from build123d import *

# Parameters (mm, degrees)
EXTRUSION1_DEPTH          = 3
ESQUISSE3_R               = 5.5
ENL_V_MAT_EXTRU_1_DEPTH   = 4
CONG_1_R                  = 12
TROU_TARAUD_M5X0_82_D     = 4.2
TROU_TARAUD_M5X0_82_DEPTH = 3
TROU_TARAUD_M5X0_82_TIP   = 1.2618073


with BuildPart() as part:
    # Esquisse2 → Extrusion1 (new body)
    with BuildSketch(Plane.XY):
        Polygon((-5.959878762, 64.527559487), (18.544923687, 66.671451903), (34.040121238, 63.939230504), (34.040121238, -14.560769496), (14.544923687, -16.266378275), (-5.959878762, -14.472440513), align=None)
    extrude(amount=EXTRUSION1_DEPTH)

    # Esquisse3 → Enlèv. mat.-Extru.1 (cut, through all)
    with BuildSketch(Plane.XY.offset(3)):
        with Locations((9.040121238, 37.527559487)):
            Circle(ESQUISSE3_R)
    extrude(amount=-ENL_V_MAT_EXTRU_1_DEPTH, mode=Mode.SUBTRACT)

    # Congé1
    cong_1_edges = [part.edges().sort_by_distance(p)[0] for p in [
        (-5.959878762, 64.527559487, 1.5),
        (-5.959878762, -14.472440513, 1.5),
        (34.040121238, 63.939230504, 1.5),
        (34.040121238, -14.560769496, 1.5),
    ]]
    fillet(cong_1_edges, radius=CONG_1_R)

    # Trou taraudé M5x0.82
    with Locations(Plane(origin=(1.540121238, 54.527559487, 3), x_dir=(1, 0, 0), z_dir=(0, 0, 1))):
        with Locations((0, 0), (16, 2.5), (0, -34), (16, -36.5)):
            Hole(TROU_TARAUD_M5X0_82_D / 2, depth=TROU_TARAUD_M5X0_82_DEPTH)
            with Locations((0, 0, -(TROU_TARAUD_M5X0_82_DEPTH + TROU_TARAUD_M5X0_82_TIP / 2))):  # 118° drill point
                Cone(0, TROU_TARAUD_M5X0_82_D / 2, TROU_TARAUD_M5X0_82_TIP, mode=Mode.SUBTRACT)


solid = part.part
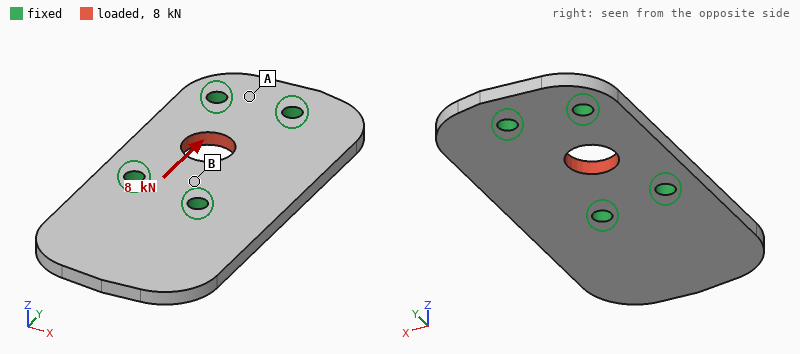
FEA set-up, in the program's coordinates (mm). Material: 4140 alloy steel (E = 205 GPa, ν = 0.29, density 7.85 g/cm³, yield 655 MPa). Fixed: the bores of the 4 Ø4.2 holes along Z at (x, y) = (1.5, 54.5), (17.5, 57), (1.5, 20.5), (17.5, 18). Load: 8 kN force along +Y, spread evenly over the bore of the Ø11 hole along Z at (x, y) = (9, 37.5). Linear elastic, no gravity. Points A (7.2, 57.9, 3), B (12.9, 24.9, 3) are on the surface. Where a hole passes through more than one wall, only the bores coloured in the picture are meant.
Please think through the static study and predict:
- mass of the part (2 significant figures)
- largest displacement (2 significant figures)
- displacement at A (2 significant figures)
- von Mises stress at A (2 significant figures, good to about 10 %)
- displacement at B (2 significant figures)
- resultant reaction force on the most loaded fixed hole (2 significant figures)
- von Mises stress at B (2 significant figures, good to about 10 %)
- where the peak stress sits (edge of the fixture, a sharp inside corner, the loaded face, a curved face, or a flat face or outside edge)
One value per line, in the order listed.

70 g
5.2 µm
0.92 µm
19 MPa
2.0 µm
2.2 kN
56 MPa
the loaded face
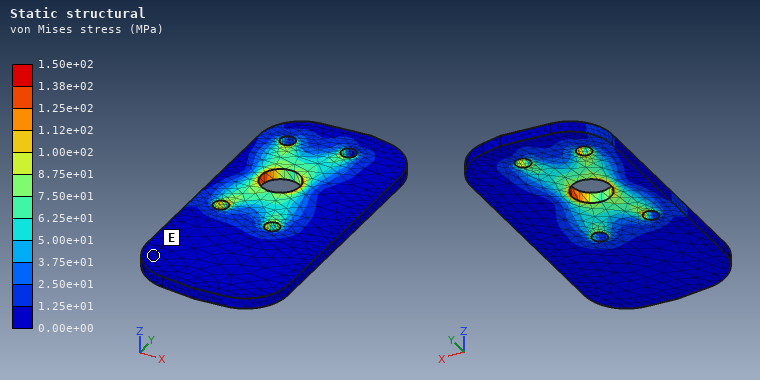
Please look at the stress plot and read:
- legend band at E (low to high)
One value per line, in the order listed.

0.00e+00 to 1.25e+01 MPa
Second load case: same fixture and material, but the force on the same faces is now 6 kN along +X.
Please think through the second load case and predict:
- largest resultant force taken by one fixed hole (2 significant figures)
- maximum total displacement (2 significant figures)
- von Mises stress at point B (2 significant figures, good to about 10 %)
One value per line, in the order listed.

1.8 kN
8.7 µm
61 MPa
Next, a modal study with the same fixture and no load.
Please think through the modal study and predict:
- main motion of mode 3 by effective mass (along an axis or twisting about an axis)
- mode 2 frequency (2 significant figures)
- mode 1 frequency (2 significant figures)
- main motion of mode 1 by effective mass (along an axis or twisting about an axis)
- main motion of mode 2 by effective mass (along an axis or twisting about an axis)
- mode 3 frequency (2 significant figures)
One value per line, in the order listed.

along Z
4700 Hz
2300 Hz
along Z
twisting about Y
7300 Hz
